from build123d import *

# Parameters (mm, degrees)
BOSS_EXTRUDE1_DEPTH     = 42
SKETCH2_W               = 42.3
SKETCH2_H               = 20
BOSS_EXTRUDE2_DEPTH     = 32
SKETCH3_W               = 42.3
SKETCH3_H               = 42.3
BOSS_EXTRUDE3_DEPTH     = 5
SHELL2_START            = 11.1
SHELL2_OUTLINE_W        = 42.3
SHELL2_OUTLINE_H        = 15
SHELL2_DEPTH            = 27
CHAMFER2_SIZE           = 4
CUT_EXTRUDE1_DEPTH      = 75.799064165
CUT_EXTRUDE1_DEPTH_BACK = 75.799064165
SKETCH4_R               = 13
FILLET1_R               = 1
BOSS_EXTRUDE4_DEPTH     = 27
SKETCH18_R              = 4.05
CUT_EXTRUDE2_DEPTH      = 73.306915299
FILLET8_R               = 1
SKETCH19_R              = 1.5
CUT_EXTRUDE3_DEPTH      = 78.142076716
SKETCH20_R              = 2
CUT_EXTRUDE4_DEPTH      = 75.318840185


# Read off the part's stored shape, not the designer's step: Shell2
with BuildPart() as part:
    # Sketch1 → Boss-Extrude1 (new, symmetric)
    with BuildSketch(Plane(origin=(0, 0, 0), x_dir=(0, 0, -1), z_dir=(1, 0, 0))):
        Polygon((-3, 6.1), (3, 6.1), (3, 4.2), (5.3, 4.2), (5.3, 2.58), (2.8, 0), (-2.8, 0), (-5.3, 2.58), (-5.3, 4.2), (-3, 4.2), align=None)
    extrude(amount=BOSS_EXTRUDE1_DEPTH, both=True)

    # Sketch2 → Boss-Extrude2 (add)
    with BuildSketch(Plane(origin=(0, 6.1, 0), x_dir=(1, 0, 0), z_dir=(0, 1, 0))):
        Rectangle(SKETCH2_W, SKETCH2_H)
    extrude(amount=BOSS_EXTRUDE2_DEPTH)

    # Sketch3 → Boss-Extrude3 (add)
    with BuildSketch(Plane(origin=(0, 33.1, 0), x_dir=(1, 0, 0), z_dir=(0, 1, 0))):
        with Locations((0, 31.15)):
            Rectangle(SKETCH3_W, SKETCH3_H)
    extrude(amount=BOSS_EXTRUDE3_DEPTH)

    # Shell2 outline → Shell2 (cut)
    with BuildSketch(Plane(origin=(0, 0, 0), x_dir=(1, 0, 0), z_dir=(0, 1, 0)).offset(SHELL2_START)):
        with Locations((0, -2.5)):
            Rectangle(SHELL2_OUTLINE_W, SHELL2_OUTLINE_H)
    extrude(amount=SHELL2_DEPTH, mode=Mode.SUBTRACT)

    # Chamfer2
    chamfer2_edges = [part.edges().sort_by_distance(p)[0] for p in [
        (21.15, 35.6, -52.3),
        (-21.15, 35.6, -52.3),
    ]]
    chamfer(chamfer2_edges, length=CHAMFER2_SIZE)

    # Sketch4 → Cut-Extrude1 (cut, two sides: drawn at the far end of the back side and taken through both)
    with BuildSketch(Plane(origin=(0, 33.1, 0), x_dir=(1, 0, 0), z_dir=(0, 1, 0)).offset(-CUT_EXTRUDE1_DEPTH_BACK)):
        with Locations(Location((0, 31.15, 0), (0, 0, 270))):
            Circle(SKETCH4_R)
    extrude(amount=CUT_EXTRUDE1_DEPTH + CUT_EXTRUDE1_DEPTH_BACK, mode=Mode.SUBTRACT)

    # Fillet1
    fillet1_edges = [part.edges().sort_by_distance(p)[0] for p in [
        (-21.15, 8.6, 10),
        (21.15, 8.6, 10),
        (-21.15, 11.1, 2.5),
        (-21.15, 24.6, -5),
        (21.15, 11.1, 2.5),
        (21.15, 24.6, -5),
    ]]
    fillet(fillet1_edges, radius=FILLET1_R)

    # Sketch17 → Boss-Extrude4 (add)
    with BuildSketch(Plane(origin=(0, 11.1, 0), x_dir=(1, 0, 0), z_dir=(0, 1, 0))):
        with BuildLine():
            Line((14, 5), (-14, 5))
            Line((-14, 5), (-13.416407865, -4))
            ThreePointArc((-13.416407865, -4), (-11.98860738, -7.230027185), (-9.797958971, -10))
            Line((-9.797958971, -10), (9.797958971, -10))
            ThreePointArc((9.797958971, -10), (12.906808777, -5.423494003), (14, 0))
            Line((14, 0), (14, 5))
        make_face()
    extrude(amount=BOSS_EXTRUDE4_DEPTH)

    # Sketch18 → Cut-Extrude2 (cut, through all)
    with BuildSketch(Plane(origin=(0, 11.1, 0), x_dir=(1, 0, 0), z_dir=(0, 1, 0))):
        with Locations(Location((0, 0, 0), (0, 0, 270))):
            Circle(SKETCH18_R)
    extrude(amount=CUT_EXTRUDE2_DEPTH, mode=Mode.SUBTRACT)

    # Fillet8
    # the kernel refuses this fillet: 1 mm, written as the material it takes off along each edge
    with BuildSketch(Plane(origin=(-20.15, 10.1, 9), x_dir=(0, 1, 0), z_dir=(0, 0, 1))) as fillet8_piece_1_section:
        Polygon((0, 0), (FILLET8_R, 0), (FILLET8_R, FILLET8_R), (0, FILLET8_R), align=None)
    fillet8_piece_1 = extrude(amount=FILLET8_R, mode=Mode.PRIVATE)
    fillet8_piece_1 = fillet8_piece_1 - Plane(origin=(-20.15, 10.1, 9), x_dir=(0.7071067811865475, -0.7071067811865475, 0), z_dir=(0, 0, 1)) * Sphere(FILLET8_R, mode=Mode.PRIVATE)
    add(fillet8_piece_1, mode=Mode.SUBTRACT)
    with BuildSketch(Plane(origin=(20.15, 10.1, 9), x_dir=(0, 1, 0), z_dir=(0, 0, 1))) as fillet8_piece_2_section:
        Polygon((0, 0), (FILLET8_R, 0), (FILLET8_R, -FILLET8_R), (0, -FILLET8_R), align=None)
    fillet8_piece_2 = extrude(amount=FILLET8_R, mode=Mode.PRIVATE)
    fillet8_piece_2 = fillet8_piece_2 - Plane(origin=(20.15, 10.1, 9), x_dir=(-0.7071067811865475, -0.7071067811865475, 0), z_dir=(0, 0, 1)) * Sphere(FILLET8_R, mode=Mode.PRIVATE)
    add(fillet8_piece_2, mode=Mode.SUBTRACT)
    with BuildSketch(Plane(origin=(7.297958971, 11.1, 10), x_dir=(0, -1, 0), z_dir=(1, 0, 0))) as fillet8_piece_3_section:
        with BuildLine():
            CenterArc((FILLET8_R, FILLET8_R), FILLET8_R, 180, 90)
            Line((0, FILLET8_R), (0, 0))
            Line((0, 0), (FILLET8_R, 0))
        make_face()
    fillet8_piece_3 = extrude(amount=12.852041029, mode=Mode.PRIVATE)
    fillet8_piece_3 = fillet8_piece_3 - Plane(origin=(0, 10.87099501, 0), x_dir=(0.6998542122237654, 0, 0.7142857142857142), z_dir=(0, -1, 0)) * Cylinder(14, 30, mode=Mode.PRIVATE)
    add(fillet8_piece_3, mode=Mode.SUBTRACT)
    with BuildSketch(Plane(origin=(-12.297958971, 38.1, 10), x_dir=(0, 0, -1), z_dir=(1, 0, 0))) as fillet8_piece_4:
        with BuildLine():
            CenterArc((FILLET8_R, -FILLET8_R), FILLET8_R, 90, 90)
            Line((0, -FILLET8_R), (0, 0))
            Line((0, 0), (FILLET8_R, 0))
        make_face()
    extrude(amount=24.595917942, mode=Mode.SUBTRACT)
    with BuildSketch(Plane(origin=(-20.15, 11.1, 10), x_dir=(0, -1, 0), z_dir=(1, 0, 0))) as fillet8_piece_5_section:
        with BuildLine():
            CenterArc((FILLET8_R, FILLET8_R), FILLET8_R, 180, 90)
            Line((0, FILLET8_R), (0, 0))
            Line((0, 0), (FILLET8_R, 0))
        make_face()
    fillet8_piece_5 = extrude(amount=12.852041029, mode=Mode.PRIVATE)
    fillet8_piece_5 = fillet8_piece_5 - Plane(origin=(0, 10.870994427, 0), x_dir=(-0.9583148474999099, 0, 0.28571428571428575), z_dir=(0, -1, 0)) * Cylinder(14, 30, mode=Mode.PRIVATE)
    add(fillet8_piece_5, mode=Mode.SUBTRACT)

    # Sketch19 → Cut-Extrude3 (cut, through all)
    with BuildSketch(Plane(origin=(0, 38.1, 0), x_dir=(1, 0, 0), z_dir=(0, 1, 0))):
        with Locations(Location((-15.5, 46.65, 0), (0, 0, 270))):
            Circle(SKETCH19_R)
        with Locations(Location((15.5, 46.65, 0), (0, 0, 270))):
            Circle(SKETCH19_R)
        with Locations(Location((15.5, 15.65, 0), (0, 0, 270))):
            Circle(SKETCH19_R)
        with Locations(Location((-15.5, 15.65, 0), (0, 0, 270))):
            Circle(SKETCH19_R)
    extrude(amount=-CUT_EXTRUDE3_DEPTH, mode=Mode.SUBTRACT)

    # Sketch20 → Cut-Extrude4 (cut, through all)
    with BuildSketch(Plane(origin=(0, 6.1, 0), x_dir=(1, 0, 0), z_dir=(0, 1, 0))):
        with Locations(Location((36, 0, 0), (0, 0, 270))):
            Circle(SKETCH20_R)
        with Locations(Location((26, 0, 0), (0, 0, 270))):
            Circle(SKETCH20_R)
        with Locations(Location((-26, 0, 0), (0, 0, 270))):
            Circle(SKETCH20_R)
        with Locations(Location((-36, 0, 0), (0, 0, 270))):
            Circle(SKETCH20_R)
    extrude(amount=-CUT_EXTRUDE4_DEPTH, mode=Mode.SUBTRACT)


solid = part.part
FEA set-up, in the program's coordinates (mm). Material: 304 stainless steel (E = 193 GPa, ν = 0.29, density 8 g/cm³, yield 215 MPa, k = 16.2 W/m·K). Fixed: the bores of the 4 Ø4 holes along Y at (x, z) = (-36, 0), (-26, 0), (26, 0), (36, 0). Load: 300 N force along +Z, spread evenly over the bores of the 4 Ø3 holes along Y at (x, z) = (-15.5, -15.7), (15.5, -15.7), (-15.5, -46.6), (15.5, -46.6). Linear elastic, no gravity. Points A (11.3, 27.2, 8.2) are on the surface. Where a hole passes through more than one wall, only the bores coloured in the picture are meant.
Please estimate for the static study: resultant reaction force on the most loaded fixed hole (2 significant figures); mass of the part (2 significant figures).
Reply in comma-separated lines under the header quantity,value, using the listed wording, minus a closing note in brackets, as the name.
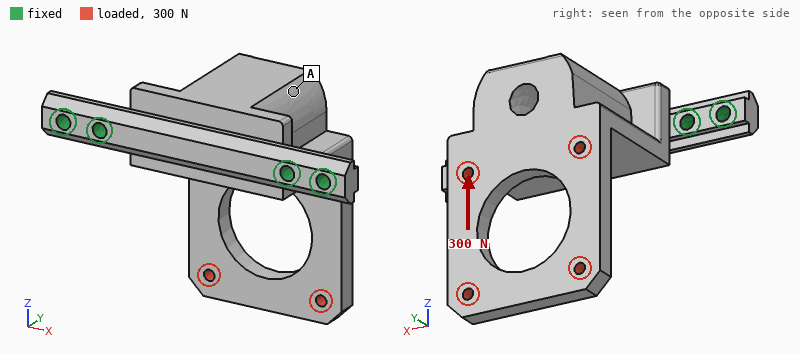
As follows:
quantity,value
resultant reaction force on the most loaded fixed hole,150 N
mass of the part,230 g
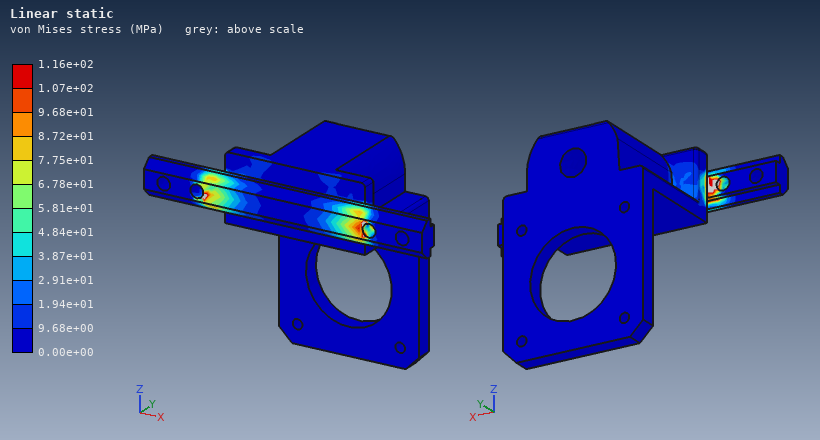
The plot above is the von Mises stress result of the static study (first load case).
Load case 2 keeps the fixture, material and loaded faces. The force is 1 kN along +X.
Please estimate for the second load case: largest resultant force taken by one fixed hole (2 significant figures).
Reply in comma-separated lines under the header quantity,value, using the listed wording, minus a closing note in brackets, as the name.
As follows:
quantity,value
largest resultant force taken by one fixed hole,1.2 kN
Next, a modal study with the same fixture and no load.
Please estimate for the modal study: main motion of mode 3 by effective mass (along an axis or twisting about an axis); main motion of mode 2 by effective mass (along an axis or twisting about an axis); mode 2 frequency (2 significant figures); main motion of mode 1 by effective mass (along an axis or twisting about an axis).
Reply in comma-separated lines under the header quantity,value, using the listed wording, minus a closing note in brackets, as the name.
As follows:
quantity,value
main motion of mode 3 by effective mass,along X
main motion of mode 2 by effective mass,along Z
mode 2 frequency,2100 Hz
main motion of mode 1 by effective mass,along Z
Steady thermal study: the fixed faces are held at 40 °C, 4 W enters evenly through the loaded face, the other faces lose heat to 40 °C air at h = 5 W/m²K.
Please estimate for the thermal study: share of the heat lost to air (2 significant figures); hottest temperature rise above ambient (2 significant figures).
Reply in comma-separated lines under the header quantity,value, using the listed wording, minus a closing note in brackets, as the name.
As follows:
quantity,value
share of the heat lost to air,37 %
hottest temperature rise above ambient,66 K
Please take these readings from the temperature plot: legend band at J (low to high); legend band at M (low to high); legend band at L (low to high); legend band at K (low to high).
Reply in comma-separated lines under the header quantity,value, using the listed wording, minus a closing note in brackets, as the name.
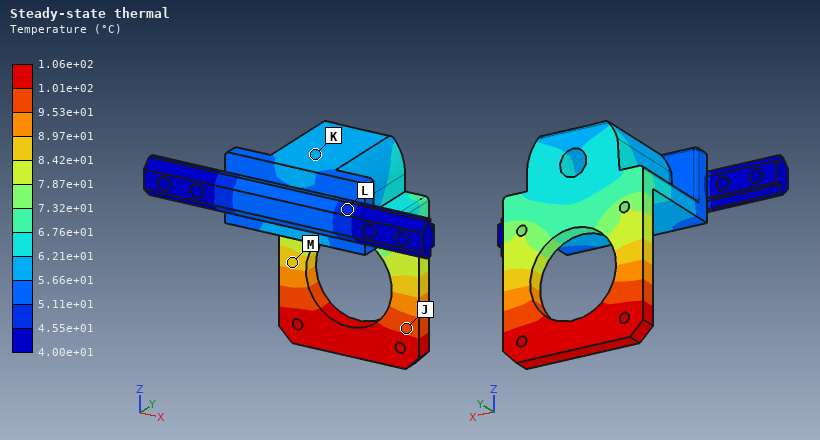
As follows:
quantity,value
legend band at J,9.53e+01 to 1.01e+02 °C
legend band at M,8.42e+01 to 8.97e+01 °C
legend band at L,4.55e+01 to 5.11e+01 °C
legend band at K,5.66e+01 to 6.21e+01 °C
